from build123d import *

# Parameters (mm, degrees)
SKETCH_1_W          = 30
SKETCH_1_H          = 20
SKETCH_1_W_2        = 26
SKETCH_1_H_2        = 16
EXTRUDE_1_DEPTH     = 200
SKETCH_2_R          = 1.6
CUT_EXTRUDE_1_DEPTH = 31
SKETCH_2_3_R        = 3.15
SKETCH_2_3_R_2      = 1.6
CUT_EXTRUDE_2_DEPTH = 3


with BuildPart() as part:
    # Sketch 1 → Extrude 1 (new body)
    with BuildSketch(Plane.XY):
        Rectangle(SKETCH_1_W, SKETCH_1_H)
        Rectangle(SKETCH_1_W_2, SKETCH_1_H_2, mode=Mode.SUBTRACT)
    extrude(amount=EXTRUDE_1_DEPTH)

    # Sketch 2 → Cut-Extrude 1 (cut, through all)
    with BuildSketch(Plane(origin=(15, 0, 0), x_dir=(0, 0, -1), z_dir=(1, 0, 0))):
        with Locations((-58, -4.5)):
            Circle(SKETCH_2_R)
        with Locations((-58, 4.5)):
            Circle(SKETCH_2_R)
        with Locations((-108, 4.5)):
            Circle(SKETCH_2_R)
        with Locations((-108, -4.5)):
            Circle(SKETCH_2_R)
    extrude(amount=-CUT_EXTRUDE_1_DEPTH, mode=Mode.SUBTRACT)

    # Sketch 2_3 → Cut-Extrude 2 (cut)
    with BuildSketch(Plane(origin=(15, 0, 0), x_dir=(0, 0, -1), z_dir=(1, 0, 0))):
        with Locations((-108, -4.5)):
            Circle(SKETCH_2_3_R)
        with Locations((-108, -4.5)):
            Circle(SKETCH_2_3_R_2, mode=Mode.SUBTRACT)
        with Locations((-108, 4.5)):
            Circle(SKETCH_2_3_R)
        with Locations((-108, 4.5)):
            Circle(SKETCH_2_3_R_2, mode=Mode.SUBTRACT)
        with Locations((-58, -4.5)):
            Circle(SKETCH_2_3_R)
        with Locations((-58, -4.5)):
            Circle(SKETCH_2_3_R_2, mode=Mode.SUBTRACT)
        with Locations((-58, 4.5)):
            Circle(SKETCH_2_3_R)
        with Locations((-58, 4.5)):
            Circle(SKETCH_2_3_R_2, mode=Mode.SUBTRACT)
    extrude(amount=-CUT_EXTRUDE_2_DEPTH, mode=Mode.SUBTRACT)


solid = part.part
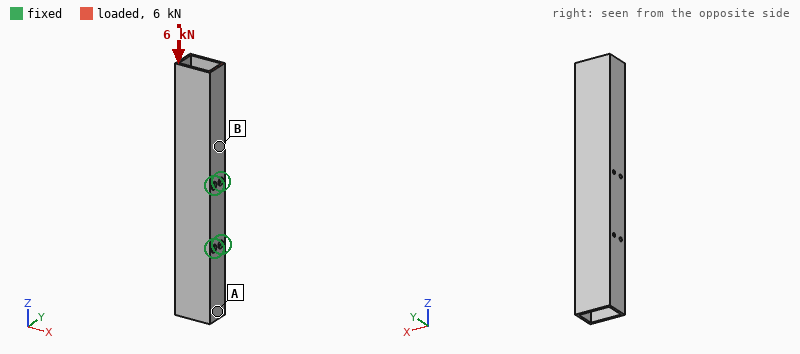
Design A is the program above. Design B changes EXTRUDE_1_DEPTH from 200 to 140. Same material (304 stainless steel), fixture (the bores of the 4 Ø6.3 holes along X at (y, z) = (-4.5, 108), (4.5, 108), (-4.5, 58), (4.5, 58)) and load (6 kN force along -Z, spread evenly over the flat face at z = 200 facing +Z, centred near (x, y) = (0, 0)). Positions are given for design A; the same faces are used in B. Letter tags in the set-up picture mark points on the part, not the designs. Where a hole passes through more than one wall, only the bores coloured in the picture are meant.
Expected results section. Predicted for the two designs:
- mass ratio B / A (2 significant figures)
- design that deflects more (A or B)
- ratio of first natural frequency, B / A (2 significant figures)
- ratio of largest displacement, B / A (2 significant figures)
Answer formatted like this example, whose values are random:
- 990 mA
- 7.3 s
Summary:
- 0.70
- A
- 1.3
- 0.49
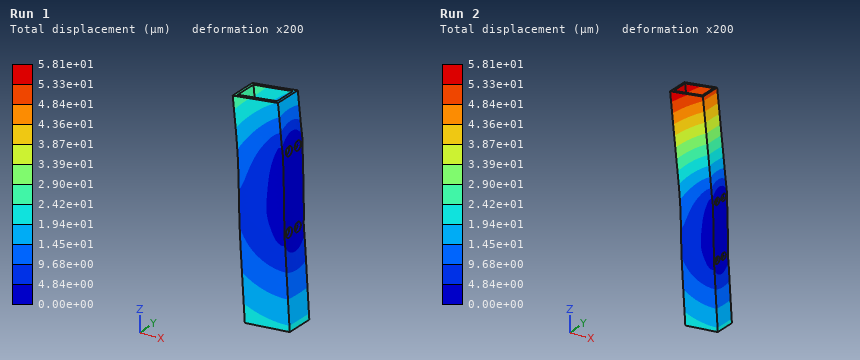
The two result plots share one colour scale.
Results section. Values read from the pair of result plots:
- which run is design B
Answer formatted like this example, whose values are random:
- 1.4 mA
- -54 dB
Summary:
- Run 1
